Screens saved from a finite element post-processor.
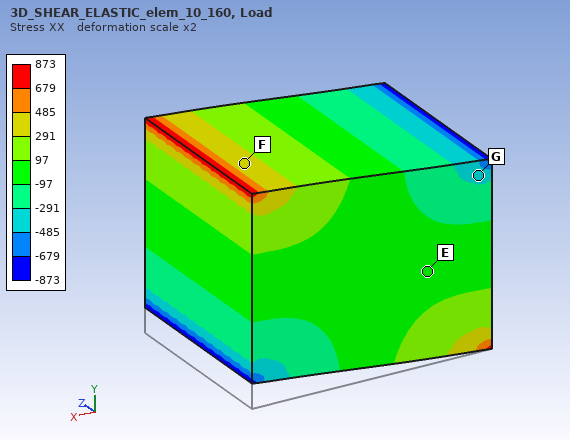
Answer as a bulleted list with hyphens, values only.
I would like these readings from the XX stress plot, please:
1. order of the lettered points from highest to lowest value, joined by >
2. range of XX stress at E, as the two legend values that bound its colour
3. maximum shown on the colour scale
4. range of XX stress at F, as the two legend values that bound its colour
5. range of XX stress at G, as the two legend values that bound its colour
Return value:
- F > E > G
- -97 to 97
- 873
- 291 to 485
- -485 to -291
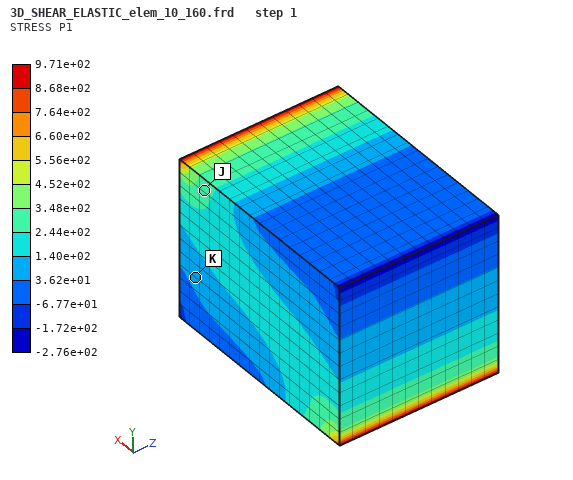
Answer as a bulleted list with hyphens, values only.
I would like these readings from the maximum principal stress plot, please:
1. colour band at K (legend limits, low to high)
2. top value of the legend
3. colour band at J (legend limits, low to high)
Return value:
- 3.62e+01 to 1.40e+02
- 9.71e+02
- 2.44e+02 to 3.48e+02
